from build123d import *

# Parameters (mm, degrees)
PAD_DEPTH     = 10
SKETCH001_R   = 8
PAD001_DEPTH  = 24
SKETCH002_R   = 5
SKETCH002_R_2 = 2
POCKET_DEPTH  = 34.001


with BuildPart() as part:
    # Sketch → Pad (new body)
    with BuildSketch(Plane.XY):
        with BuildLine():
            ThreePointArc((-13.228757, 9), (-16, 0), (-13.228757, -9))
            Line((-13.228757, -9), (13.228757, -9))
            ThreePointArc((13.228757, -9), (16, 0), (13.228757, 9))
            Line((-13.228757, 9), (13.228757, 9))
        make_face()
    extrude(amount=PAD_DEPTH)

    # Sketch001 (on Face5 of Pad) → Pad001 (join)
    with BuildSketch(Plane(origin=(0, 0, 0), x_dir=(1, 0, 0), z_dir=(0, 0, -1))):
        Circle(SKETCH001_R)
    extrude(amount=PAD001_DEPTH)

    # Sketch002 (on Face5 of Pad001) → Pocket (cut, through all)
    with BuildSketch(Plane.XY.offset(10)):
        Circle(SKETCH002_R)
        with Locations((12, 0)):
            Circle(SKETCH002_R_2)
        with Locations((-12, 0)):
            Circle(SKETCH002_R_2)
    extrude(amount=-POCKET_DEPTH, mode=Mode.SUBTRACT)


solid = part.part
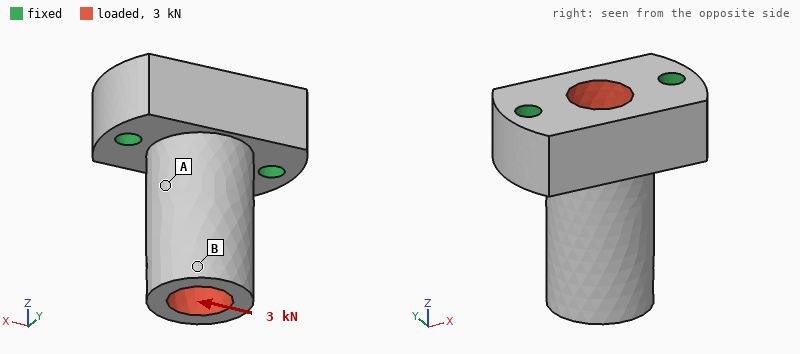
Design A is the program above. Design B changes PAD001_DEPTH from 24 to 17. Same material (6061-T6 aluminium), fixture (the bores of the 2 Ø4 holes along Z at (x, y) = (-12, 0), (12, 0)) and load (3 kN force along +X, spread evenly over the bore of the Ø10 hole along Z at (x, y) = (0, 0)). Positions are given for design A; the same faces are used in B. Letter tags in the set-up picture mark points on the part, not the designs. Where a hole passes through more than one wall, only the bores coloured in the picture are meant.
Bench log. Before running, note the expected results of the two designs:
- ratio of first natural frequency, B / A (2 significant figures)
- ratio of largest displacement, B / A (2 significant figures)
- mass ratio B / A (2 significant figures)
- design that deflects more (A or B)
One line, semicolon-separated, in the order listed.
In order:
1.5; 0.48; 0.88; A
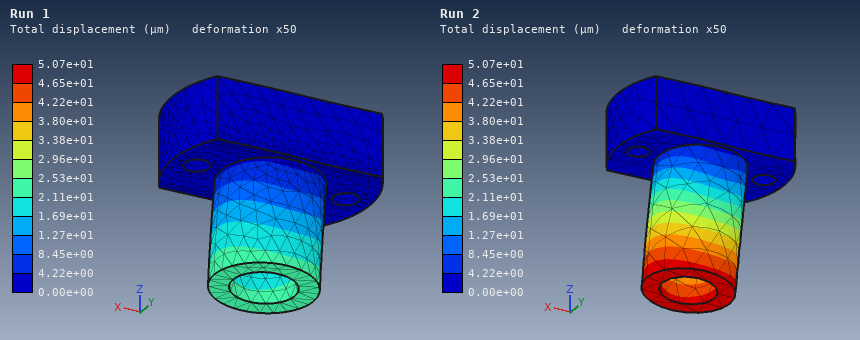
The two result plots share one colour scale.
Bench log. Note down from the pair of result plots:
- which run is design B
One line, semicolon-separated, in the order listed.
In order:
Run 1
